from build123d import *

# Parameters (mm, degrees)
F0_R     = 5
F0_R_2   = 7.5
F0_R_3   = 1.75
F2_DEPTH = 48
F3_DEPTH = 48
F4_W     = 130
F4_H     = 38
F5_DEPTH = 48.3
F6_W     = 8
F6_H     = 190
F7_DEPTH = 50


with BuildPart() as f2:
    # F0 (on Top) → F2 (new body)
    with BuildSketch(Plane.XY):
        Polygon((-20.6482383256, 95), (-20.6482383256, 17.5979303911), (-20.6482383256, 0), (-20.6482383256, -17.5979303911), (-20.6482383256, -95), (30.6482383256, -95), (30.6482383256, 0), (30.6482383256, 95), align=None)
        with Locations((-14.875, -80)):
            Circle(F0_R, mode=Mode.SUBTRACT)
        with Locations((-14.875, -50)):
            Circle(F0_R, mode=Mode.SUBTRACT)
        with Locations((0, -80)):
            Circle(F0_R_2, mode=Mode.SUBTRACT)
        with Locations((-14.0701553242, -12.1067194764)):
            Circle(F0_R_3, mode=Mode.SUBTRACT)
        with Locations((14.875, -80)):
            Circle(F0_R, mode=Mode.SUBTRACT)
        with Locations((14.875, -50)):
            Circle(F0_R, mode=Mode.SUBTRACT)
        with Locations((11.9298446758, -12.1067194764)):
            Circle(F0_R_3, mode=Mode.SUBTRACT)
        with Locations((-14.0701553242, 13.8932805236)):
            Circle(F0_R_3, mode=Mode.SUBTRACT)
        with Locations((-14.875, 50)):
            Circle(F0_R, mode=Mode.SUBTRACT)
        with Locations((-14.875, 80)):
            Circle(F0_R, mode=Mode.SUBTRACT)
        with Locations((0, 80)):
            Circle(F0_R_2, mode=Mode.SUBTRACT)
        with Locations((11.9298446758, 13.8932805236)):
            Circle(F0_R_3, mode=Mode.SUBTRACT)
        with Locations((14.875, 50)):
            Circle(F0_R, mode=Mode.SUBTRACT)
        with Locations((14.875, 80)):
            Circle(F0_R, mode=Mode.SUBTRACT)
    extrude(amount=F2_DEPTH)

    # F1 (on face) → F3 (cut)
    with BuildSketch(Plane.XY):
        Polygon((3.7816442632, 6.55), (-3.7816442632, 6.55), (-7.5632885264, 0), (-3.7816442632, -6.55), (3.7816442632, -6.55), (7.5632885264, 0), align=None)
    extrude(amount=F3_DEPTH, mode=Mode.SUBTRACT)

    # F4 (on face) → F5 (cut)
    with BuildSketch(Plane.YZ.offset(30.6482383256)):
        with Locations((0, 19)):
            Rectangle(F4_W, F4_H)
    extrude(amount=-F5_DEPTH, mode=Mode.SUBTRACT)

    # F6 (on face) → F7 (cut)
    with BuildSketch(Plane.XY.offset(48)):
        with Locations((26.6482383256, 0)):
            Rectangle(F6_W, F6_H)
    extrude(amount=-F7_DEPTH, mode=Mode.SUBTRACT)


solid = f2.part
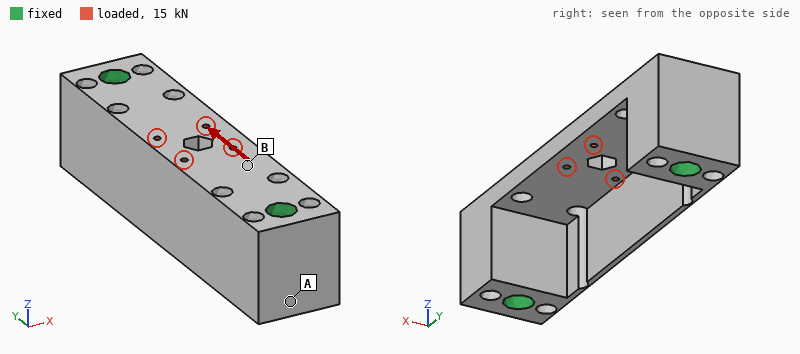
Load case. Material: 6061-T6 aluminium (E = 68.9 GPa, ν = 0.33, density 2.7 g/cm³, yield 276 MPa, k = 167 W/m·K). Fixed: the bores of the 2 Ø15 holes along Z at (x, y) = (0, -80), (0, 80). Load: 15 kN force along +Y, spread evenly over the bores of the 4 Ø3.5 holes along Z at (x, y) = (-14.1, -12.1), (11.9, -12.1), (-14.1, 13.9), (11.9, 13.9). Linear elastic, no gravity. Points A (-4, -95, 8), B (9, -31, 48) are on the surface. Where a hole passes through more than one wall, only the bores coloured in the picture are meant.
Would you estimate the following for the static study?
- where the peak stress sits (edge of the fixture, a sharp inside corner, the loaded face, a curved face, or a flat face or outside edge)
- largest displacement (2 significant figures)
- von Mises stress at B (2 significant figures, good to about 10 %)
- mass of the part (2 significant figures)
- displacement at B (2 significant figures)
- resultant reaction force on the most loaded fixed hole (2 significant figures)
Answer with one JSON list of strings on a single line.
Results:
["a curved face", "21 µm", "17 MPa", "430 g", "14 µm", "7.6 kN"]
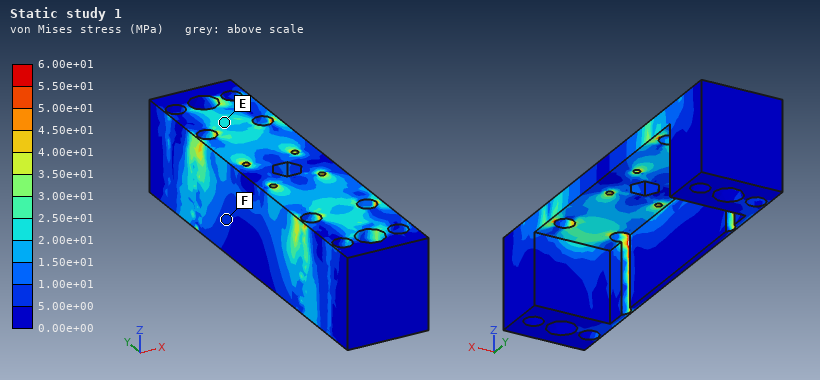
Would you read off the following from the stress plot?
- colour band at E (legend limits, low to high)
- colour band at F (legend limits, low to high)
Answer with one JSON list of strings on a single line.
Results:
["2.00e+01 to 2.50e+01 MPa", "5.00e+00 to 1.00e+01 MPa"]
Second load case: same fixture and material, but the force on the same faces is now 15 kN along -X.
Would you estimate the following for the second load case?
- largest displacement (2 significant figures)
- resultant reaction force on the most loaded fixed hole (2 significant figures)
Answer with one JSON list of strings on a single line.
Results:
["0.14 mm", "7.6 kN"]
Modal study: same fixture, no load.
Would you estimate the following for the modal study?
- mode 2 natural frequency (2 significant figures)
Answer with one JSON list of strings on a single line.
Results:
["3400 Hz"]
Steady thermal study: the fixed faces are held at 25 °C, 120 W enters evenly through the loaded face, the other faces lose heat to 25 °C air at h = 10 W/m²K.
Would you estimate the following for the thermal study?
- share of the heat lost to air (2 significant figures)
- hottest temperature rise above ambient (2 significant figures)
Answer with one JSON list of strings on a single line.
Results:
["6.0 %", "51 K"]
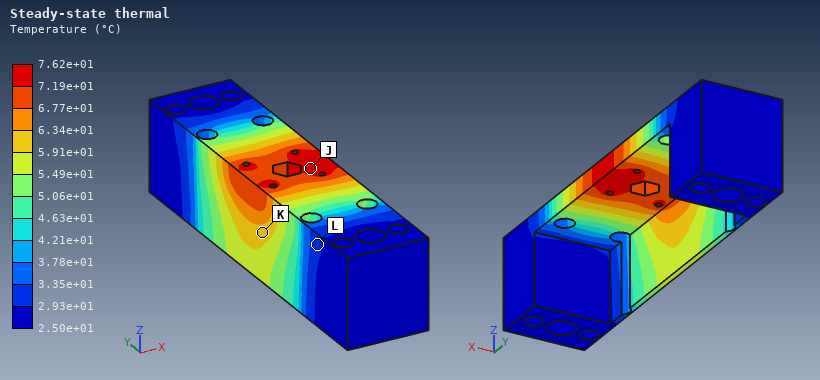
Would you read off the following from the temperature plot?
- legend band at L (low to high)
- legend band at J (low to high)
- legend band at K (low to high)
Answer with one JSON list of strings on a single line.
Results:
["2.93e+01 to 3.35e+01 °C", "7.19e+01 to 7.62e+01 °C", "5.91e+01 to 6.34e+01 °C"]
